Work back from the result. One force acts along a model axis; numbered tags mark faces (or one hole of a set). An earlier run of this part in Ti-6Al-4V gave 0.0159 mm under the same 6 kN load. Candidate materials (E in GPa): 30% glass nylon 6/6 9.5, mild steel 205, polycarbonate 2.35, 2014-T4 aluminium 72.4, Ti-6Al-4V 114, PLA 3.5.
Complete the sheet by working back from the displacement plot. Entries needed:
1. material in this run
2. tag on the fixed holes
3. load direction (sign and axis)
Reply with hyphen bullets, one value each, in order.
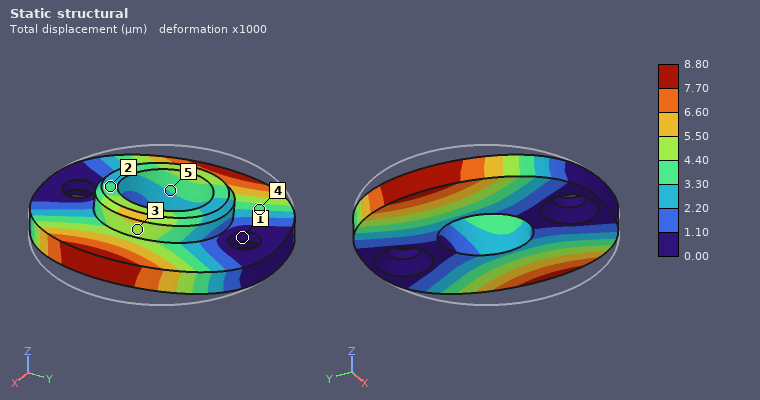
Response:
- mild steel
- 1
- -X
